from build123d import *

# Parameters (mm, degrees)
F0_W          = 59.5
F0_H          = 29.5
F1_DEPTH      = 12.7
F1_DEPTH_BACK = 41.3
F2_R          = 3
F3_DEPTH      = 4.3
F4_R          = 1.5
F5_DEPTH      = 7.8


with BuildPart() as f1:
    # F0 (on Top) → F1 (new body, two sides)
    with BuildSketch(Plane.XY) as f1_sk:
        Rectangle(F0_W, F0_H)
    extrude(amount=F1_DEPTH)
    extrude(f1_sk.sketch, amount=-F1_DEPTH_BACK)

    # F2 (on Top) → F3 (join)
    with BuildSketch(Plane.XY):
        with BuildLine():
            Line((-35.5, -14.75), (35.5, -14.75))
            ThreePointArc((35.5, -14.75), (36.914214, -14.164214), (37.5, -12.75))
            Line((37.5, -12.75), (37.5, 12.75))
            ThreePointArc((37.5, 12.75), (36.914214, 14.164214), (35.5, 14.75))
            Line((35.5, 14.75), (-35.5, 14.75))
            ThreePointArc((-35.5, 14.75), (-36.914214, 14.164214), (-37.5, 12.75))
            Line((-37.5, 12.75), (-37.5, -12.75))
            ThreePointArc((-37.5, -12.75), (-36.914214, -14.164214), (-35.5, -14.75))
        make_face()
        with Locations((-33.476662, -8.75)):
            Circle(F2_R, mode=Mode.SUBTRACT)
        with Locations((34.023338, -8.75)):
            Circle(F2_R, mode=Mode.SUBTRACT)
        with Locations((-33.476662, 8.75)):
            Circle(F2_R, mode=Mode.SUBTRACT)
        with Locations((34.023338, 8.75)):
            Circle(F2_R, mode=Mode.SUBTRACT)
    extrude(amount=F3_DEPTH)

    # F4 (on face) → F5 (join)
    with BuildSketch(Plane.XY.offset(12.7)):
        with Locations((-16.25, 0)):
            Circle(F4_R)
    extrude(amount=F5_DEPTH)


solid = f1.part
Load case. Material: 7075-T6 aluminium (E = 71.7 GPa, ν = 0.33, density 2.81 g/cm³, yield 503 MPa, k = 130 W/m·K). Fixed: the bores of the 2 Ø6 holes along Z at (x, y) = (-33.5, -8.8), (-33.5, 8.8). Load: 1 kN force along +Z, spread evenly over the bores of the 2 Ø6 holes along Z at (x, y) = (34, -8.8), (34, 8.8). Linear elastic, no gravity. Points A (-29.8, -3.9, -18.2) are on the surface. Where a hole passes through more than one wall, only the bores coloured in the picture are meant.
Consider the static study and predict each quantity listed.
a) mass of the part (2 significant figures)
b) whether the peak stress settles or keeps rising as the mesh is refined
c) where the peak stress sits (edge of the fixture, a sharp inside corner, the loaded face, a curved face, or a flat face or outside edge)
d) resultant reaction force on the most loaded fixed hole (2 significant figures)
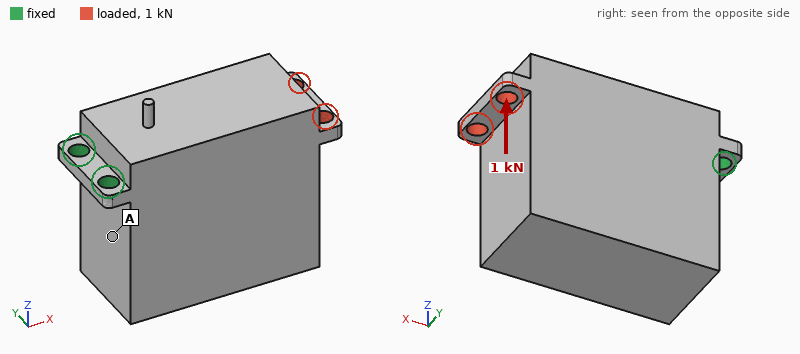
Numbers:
270 g
keeps rising
edge of the fixture
500 N
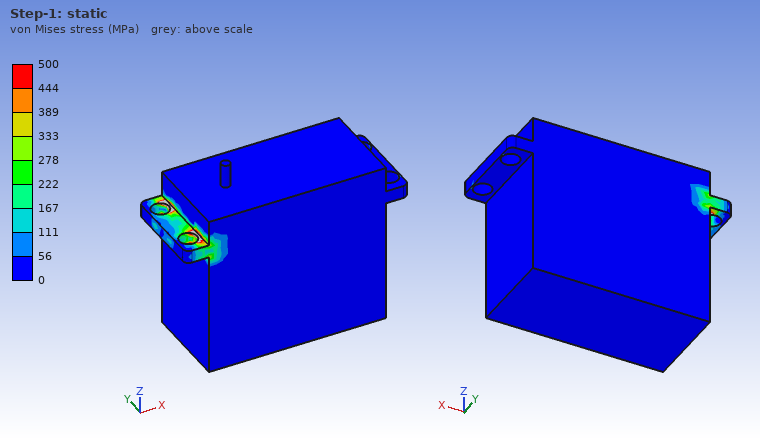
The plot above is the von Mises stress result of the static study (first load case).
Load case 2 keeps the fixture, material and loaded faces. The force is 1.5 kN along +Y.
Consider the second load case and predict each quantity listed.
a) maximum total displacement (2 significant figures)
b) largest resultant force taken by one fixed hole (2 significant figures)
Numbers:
0.11 mm
5.0 kN
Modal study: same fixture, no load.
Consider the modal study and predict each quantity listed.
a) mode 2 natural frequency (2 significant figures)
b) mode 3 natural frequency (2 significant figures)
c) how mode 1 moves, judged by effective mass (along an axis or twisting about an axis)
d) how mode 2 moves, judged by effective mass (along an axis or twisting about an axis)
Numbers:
2000 Hz
3600 Hz
along Z
along Y
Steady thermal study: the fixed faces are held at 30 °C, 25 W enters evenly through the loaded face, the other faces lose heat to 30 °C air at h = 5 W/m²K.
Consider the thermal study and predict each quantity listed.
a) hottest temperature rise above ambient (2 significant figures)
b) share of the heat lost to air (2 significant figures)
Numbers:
38 K
3.4 %
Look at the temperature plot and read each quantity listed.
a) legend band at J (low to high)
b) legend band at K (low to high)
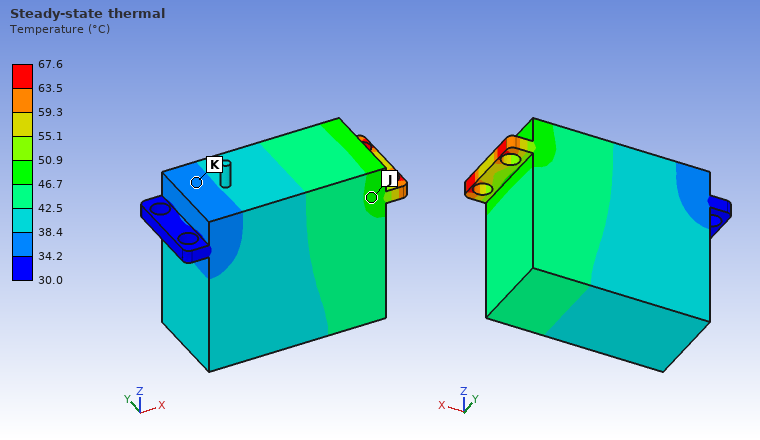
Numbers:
46.7 to 50.9 °C
34.2 to 38.4 °C
